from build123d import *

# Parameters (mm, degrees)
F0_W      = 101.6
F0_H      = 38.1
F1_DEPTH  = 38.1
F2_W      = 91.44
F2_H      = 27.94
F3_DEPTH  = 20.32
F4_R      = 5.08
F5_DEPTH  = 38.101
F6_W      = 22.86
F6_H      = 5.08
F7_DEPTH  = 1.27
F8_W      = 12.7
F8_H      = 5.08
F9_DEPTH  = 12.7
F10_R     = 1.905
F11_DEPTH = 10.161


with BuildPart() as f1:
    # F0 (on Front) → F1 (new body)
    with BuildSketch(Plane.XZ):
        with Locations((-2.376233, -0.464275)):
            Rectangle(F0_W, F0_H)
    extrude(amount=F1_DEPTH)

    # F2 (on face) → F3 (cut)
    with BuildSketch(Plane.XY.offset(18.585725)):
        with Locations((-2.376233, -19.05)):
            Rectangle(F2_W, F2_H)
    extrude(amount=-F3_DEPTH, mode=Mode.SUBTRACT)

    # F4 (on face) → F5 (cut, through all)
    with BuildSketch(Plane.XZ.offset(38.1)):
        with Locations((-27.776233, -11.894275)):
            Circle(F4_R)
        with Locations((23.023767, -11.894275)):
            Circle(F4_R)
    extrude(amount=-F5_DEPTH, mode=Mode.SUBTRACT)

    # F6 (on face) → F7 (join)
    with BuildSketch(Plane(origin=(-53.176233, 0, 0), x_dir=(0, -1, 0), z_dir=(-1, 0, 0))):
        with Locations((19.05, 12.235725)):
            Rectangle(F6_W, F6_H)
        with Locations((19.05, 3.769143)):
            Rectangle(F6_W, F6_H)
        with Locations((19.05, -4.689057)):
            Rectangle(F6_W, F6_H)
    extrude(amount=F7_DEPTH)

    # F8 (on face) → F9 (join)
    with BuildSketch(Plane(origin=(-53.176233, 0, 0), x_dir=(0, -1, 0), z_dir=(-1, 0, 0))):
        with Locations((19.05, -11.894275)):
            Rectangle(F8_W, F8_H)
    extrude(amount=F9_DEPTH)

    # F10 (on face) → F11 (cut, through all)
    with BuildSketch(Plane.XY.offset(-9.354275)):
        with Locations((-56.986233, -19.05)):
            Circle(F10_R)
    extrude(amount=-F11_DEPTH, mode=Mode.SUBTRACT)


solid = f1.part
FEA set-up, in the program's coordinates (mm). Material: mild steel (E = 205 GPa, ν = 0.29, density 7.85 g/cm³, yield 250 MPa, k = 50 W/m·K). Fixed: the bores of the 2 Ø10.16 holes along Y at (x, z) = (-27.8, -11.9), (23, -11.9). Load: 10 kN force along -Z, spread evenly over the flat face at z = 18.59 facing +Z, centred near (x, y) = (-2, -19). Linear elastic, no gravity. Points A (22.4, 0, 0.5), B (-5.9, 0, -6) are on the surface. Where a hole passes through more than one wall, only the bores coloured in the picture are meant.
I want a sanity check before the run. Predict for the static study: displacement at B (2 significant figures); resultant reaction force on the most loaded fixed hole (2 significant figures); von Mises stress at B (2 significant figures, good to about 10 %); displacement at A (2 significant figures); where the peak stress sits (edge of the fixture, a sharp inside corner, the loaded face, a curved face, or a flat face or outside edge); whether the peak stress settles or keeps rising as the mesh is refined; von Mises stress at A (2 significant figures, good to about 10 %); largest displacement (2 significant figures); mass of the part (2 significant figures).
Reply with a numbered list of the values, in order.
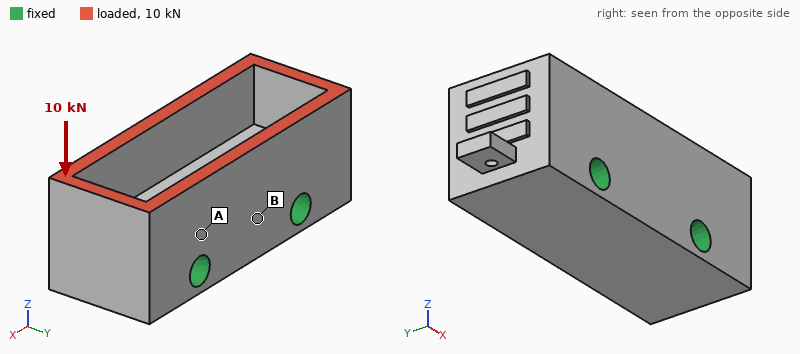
1. 0.59 µm
2. 5.0 kN
3. 3.9 MPa
4. 0.64 µm
5. edge of the fixture
6. keeps rising
7. 13 MPa
8. 3.2 µm
9. 710 g
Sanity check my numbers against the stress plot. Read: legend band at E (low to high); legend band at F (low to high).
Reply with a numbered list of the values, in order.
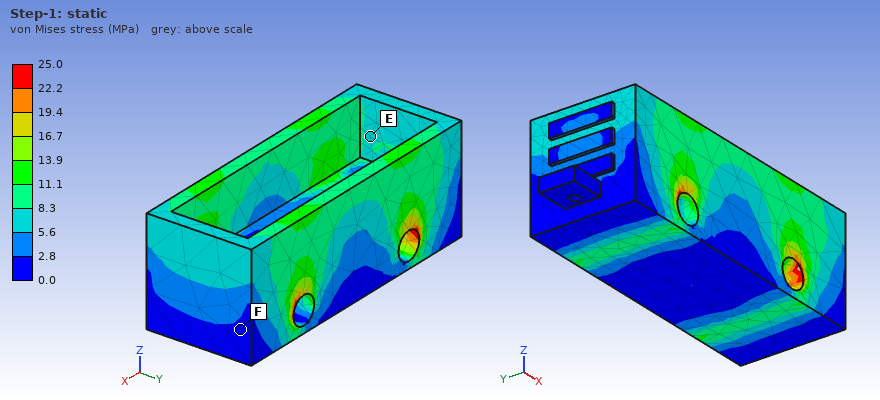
1. 5.6 to 8.3 MPa
2. 0.0 to 2.8 MPa
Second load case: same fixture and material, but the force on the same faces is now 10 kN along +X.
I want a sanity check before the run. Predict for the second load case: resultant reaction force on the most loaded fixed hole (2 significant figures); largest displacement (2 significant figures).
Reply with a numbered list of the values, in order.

1. 6.3 kN
2. 19 µm
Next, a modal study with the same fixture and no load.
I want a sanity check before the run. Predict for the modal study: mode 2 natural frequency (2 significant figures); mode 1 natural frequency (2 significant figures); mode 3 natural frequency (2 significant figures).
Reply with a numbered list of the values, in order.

1. 9000 Hz
2. 9000 Hz
3. 11 kHz
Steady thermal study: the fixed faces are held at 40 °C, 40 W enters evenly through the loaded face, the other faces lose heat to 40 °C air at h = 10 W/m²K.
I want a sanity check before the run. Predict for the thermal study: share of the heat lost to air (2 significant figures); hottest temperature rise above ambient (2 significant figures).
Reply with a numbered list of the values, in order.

1. 3.6 %
2. 18 K
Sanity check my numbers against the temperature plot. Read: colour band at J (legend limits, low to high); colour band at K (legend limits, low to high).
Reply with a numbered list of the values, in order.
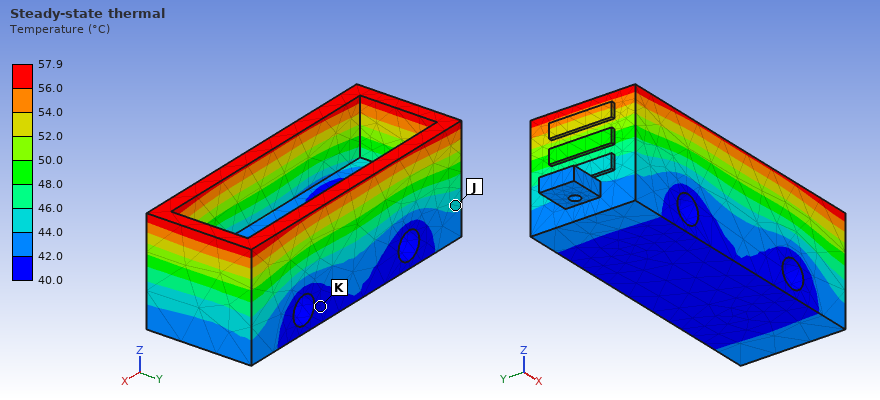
1. 44.0 to 46.0 °C
2. 40.0 to 42.0 °C
